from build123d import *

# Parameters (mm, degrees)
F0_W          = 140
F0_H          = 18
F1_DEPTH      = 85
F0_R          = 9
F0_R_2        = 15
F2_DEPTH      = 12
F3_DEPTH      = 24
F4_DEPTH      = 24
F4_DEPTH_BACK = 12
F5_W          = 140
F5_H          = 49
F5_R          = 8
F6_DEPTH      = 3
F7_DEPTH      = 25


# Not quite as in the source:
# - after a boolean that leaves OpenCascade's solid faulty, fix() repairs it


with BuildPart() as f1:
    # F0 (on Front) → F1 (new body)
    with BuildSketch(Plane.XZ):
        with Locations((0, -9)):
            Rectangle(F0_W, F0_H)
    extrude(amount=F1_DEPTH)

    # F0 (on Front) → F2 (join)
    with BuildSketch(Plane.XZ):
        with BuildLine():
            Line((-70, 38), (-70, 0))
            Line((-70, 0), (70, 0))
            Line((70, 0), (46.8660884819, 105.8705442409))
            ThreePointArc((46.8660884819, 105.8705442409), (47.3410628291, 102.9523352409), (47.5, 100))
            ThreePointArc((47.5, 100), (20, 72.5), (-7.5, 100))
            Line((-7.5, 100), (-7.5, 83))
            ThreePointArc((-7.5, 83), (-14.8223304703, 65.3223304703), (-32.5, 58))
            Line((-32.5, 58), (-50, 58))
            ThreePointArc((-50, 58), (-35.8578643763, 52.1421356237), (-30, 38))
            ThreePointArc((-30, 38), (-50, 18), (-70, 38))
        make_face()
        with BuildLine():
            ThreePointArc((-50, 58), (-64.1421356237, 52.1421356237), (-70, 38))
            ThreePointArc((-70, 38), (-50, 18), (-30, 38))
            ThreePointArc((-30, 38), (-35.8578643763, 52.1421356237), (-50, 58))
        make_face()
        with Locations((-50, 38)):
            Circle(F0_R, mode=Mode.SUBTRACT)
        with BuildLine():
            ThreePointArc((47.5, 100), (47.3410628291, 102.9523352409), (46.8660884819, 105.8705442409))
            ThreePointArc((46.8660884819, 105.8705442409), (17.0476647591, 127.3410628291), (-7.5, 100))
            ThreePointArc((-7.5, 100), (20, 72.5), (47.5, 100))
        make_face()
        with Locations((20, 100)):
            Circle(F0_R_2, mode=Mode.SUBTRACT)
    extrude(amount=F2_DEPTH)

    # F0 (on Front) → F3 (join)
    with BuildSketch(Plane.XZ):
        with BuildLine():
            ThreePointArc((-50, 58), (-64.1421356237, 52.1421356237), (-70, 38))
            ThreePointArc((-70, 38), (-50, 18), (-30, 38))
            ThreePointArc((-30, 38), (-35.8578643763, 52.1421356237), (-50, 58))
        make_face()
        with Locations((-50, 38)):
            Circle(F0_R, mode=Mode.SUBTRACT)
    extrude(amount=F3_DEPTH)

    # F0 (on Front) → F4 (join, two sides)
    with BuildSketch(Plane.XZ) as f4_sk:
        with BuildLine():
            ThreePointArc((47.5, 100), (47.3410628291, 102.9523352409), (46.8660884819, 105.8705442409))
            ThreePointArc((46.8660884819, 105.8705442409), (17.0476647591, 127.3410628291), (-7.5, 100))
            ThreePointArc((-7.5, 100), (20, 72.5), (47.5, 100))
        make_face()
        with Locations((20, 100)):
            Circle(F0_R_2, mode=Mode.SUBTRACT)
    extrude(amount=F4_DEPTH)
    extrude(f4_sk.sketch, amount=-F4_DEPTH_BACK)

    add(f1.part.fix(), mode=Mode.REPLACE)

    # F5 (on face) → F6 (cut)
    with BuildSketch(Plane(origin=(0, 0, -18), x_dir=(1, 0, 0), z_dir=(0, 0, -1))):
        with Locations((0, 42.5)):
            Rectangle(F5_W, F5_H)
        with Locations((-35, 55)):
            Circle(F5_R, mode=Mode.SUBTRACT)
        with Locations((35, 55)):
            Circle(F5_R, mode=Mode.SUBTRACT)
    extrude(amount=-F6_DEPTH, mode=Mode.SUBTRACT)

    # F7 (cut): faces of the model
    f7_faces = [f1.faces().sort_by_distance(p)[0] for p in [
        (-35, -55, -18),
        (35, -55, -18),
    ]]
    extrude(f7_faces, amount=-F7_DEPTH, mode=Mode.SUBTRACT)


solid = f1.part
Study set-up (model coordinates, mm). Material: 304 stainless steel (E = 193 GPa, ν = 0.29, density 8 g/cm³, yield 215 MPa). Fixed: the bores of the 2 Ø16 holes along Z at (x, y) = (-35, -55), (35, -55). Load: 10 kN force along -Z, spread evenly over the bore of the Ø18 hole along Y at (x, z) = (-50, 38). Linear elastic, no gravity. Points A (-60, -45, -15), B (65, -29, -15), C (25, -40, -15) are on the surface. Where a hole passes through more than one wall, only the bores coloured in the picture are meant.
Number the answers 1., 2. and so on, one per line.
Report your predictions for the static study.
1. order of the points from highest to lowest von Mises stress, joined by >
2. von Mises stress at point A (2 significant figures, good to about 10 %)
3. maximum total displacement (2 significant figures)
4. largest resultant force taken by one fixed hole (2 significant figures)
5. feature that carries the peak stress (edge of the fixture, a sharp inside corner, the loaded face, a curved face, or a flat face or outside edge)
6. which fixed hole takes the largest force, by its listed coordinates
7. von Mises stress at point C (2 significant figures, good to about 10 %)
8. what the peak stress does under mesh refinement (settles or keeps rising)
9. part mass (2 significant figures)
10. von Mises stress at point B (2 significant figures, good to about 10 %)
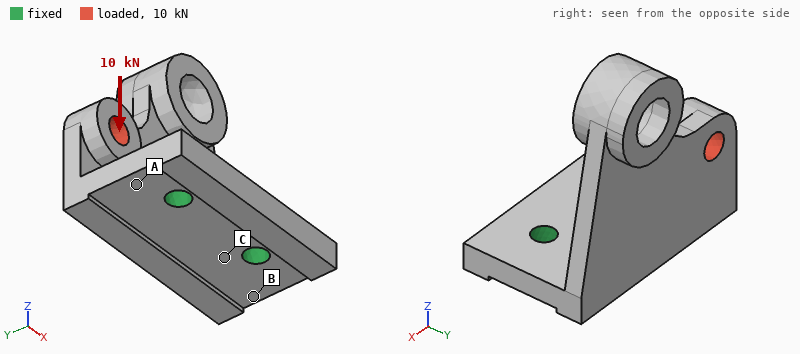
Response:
1. A > C > B
2. 69 MPa
3. 0.14 mm
4. 11 kN
5. edge of the fixture
6. (-35, -55)
7. 42 MPa
8. keeps rising
9. 2.9 kg
10. 22 MPa
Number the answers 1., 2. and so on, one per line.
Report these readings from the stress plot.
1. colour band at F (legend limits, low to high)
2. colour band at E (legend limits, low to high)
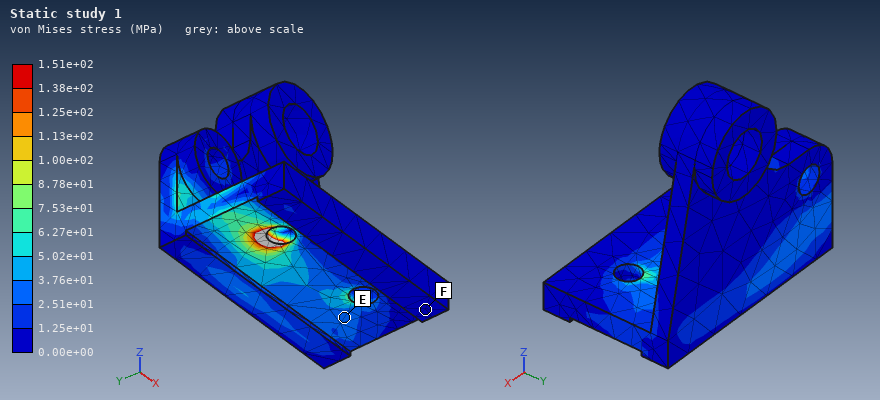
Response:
1. 0.00e+00 to 1.25e+01 MPa
2. 2.51e+01 to 3.76e+01 MPa
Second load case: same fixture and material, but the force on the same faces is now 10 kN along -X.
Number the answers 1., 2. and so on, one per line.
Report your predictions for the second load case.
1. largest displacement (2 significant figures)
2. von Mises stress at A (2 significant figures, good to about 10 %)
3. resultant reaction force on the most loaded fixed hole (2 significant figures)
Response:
1. 0.12 mm
2. 37 MPa
3. 8.8 kN
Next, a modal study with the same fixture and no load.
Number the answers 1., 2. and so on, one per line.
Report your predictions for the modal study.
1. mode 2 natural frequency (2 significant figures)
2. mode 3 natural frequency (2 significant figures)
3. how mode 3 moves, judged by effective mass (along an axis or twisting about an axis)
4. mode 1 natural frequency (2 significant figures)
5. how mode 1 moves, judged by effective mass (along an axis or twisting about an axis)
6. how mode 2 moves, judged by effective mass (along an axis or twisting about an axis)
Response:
1. 1200 Hz
2. 1700 Hz
3. along Z
4. 470 Hz
5. along Y
6. along X
